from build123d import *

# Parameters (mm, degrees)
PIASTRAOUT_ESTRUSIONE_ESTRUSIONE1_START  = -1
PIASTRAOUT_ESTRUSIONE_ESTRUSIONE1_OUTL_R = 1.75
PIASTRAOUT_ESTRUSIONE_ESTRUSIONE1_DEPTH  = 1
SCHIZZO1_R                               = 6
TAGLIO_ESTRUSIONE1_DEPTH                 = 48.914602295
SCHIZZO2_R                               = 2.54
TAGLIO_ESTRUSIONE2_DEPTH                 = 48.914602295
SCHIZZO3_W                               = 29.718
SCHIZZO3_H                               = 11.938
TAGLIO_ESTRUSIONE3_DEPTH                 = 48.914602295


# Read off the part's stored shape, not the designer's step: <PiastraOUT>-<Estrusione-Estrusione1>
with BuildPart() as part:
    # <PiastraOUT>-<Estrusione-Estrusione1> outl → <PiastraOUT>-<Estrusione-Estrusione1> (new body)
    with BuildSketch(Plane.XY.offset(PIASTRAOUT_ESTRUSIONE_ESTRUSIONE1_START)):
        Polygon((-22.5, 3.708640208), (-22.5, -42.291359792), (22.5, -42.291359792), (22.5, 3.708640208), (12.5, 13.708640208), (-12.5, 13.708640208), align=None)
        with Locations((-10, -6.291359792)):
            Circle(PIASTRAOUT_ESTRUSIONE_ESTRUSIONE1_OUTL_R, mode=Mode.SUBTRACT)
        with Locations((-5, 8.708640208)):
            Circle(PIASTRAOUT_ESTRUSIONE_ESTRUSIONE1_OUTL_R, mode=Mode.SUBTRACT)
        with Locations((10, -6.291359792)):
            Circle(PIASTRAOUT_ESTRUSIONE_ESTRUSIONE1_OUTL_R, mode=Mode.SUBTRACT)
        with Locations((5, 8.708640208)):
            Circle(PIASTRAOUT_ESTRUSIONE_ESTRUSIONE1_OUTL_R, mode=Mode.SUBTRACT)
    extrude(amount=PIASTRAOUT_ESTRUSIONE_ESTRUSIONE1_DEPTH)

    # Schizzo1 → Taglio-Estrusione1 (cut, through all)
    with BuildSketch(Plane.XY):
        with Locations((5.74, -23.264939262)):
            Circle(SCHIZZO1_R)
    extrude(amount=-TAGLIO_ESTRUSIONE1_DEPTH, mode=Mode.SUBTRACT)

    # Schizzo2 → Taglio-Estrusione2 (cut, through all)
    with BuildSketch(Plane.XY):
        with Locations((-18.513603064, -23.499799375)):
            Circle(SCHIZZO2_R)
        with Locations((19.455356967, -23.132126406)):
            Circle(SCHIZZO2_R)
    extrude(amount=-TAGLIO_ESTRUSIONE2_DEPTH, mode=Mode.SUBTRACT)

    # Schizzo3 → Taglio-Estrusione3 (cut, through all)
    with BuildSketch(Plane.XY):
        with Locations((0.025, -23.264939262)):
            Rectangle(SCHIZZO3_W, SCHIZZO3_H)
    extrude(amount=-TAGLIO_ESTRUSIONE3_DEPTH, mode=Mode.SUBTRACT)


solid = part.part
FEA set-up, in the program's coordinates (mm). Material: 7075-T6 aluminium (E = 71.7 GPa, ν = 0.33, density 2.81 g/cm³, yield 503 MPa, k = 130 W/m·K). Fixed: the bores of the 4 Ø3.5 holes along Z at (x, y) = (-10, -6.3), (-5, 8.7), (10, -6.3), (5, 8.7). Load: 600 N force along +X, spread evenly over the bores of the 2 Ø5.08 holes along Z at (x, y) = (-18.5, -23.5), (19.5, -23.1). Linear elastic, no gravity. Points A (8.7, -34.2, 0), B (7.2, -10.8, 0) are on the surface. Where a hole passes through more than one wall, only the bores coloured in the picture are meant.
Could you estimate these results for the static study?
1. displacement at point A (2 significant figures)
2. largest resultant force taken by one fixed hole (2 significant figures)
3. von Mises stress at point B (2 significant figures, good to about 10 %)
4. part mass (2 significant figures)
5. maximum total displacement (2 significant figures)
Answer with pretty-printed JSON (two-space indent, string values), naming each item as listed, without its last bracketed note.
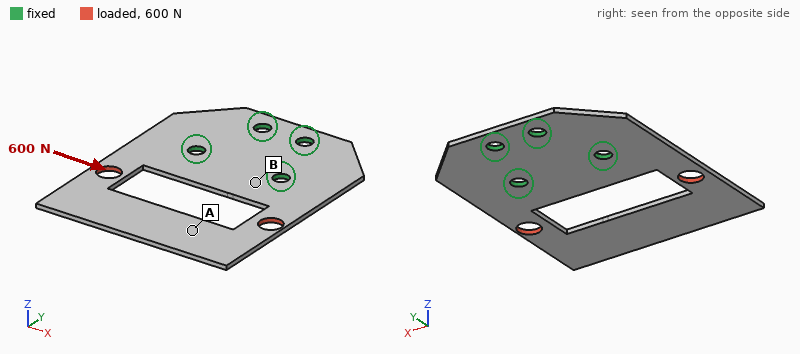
{
  "displacement at point A": "0.12 mm",
  "largest resultant force taken by one fixed hole": "480 N",
  "von Mises stress at point B": "49 MPa",
  "part mass": "5.6 g",
  "maximum total displacement": "0.13 mm"
}
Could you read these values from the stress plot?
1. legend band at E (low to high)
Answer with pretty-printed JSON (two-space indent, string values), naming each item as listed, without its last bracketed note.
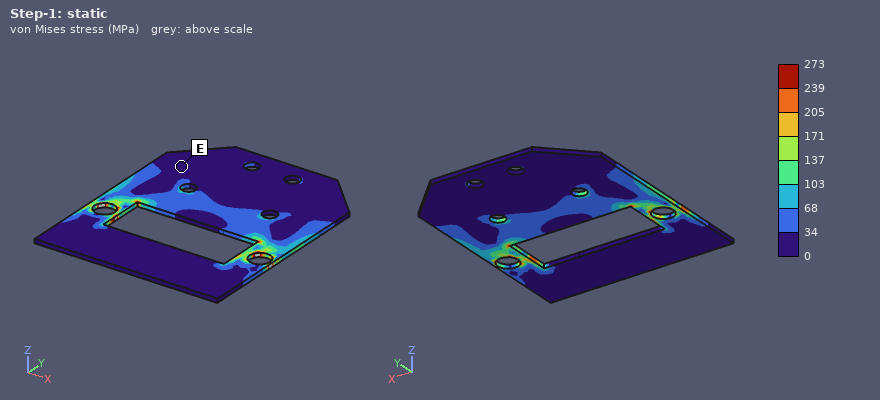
{
  "legend band at E": "0 to 34 MPa"
}
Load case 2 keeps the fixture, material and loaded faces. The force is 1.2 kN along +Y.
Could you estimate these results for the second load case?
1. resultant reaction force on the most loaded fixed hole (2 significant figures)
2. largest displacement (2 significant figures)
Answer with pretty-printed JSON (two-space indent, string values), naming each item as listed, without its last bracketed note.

{
  "resultant reaction force on the most loaded fixed hole": "510 N",
  "largest displacement": "38 µm"
}
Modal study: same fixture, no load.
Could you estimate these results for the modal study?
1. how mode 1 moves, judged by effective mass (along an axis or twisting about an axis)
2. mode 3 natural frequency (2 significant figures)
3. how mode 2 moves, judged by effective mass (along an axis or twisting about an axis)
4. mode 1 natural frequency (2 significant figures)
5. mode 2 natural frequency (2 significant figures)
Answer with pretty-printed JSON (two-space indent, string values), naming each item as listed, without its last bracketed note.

{
  "how mode 1 moves, judged by effective mass": "along Z",
  "mode 3 natural frequency": "2800 Hz",
  "how mode 2 moves, judged by effective mass": "twisting about Y",
  "mode 1 natural frequency": "430 Hz",
  "mode 2 natural frequency": "1100 Hz"
}
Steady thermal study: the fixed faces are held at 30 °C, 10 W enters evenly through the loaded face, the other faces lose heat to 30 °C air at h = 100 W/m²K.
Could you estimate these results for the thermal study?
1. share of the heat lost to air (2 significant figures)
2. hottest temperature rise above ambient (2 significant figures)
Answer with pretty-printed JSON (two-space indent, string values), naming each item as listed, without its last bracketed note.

{
  "share of the heat lost to air": "53 %",
  "hottest temperature rise above ambient": "47 K"
}
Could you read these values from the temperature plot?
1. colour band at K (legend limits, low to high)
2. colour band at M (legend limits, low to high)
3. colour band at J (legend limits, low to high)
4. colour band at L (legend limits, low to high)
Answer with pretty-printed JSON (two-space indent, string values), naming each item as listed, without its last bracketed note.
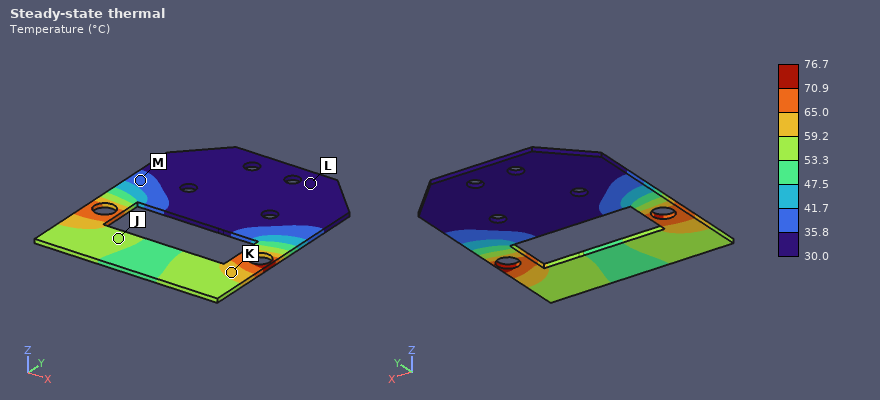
{
  "colour band at K": "59.2 to 65.0 °C",
  "colour band at M": "35.8 to 41.7 °C",
  "colour band at J": "53.3 to 59.2 °C",
  "colour band at L": "30.0 to 35.8 °C"
}
